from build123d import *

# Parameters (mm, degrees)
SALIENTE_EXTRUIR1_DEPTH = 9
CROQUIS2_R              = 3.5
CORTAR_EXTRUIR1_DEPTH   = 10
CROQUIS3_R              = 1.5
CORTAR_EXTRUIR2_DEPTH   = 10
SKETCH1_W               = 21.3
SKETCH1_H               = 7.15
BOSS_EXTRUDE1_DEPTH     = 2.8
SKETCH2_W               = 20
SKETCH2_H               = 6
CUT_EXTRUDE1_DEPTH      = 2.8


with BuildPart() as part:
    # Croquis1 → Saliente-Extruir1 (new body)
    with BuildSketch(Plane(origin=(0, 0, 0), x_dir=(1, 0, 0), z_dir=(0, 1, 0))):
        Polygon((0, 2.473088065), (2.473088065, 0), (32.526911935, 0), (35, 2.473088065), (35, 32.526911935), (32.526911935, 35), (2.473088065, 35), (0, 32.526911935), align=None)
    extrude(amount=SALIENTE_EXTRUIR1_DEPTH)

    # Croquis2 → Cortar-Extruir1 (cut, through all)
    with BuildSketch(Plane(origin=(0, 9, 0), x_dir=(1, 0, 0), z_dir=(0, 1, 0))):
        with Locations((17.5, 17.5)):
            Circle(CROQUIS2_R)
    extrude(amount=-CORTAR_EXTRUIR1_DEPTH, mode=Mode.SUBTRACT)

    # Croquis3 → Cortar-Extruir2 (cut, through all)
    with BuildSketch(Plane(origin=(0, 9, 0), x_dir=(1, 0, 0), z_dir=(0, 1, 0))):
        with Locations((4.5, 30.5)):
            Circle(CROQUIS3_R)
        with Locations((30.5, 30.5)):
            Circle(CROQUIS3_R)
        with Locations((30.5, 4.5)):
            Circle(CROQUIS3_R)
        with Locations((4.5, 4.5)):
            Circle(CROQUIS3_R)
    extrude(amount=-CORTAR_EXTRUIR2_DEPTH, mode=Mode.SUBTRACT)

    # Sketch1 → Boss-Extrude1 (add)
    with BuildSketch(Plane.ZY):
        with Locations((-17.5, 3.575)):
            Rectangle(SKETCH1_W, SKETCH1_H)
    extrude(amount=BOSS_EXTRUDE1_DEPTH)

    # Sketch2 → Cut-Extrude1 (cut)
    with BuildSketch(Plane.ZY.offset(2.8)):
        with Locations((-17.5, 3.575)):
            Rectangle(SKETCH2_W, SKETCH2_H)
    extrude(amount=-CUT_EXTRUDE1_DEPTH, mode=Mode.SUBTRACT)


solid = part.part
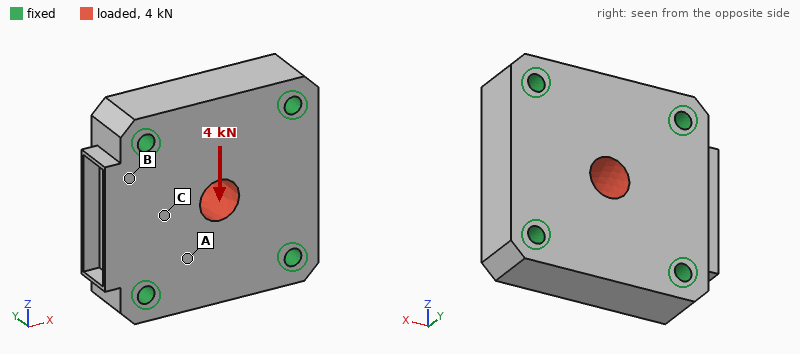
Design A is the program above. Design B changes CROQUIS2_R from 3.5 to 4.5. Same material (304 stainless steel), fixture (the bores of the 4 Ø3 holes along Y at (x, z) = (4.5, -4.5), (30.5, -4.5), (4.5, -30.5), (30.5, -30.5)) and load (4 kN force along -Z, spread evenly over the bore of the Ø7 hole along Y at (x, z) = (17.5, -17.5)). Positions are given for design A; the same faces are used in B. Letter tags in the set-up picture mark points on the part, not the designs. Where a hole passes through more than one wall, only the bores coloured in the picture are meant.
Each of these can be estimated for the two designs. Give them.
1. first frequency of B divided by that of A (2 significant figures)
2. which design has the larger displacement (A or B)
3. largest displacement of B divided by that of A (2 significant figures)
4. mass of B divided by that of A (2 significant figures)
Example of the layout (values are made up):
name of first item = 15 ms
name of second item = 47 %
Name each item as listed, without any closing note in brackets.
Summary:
first frequency of B divided by that of A = 1.0
which design has the larger displacement = A
largest displacement of B divided by that of A = 0.92
mass of B divided by that of A = 0.98
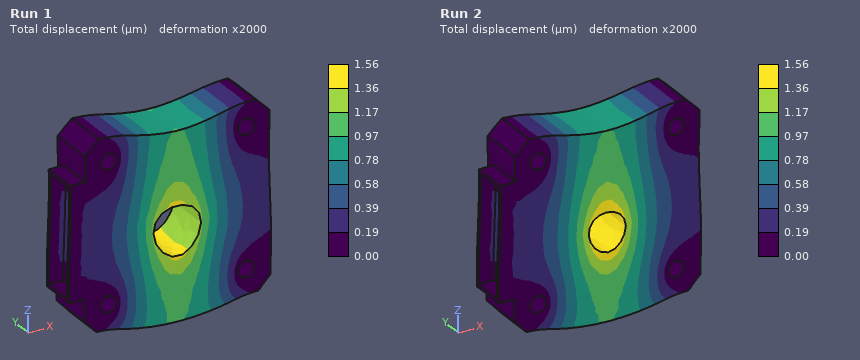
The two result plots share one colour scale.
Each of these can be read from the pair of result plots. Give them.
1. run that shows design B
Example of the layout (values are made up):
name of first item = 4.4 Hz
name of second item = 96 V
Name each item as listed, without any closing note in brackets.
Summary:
run that shows design B = Run 1
